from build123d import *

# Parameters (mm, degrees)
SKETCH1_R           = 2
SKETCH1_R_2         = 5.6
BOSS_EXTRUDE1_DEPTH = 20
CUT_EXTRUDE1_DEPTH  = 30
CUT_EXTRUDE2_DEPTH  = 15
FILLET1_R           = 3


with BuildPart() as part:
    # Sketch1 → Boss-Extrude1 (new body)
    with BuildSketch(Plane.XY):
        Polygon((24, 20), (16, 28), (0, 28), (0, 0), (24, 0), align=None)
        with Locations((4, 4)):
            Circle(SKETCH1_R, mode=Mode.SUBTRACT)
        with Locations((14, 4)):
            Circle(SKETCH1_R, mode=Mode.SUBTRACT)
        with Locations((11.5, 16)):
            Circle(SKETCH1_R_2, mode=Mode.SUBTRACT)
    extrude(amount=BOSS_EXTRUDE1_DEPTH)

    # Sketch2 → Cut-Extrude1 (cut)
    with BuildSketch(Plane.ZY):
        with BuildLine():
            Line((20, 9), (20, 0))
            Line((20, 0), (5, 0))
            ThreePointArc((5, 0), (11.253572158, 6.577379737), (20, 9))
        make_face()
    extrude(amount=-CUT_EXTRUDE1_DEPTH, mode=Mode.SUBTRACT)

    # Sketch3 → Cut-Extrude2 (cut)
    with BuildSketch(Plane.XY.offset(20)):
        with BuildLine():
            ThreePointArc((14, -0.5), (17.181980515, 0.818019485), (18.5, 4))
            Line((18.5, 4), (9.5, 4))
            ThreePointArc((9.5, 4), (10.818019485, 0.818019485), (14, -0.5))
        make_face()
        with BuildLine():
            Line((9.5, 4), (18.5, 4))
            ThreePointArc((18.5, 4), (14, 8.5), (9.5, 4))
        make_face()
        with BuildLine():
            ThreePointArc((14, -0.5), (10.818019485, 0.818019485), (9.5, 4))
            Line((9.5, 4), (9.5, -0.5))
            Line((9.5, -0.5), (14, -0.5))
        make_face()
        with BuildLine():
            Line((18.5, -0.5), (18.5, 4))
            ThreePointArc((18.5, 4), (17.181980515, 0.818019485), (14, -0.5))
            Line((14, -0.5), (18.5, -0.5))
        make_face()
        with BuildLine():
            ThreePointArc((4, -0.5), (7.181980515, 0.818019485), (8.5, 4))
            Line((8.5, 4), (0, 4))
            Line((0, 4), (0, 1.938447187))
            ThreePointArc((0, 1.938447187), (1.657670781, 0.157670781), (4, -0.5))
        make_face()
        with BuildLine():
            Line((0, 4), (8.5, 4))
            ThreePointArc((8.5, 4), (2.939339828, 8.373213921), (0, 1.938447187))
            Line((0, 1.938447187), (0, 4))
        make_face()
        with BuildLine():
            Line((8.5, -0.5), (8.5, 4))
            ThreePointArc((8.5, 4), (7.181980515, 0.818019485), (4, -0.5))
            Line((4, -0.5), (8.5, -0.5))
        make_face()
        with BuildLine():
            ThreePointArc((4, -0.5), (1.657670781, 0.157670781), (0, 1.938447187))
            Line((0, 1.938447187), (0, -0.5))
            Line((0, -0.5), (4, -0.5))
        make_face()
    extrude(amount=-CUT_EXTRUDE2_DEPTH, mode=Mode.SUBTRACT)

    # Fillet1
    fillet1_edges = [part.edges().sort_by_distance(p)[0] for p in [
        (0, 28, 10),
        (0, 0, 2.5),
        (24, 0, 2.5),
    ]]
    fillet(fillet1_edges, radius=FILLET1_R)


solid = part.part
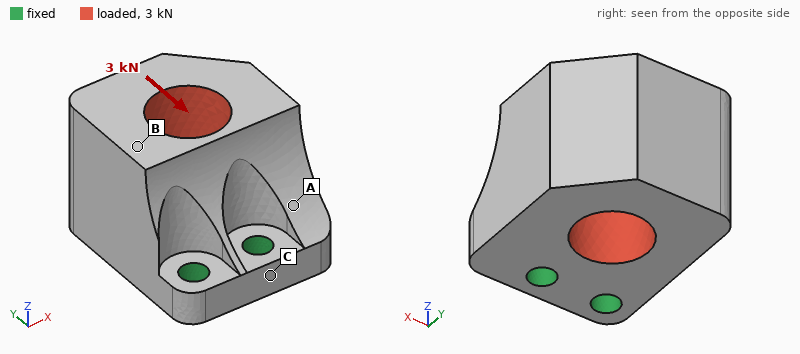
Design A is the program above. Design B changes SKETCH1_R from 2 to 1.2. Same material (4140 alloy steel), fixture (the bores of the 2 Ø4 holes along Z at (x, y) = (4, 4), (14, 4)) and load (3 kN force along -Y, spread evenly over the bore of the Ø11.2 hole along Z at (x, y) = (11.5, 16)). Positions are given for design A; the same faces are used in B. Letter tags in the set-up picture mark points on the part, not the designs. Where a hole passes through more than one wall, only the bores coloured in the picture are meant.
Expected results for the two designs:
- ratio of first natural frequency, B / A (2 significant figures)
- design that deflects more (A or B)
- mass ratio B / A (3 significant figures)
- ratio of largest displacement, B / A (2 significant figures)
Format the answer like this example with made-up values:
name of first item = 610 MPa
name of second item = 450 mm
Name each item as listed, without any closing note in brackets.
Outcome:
ratio of first natural frequency, B / A = 0.86
design that deflects more = B
mass ratio B / A = 1.01
ratio of largest displacement, B / A = 1.3
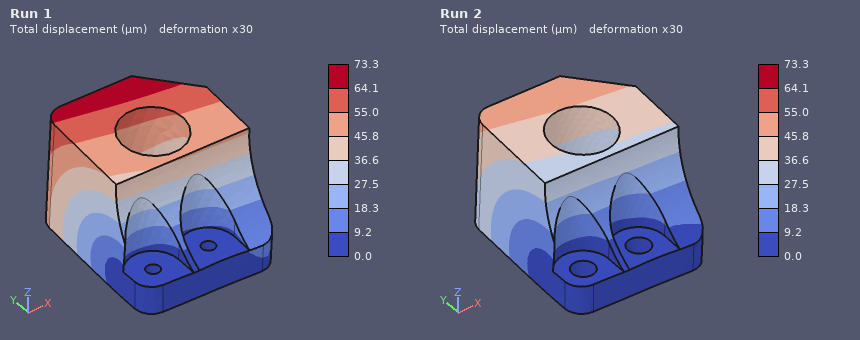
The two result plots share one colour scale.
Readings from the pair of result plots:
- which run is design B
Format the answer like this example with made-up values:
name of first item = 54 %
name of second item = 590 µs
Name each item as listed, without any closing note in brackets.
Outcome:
which run is design B = Run 1
